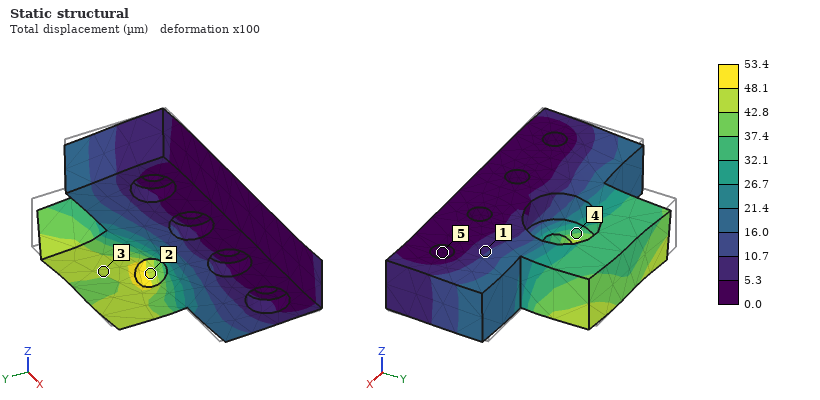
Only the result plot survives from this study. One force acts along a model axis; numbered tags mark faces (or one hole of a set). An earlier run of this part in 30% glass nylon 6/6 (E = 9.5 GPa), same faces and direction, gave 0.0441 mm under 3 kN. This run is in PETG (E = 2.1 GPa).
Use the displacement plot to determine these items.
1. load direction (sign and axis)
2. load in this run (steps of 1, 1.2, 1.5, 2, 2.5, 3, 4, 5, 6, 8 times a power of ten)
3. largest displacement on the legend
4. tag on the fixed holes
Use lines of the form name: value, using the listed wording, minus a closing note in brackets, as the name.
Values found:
load direction: +X
load in this run: 800 N
largest displacement on the legend: 53.4 µm
tag on the fixed holes: 5
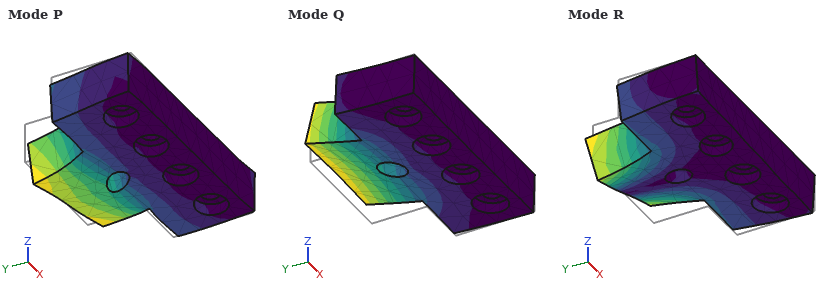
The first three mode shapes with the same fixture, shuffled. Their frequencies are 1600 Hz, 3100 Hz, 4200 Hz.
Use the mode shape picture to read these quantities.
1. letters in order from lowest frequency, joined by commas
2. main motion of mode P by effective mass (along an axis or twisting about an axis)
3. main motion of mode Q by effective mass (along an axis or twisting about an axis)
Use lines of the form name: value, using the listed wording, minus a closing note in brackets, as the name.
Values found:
letters in order from lowest frequency, joined by commas: Q, R, P
main motion of mode P by effective mass: along X
main motion of mode Q by effective mass: along Z
